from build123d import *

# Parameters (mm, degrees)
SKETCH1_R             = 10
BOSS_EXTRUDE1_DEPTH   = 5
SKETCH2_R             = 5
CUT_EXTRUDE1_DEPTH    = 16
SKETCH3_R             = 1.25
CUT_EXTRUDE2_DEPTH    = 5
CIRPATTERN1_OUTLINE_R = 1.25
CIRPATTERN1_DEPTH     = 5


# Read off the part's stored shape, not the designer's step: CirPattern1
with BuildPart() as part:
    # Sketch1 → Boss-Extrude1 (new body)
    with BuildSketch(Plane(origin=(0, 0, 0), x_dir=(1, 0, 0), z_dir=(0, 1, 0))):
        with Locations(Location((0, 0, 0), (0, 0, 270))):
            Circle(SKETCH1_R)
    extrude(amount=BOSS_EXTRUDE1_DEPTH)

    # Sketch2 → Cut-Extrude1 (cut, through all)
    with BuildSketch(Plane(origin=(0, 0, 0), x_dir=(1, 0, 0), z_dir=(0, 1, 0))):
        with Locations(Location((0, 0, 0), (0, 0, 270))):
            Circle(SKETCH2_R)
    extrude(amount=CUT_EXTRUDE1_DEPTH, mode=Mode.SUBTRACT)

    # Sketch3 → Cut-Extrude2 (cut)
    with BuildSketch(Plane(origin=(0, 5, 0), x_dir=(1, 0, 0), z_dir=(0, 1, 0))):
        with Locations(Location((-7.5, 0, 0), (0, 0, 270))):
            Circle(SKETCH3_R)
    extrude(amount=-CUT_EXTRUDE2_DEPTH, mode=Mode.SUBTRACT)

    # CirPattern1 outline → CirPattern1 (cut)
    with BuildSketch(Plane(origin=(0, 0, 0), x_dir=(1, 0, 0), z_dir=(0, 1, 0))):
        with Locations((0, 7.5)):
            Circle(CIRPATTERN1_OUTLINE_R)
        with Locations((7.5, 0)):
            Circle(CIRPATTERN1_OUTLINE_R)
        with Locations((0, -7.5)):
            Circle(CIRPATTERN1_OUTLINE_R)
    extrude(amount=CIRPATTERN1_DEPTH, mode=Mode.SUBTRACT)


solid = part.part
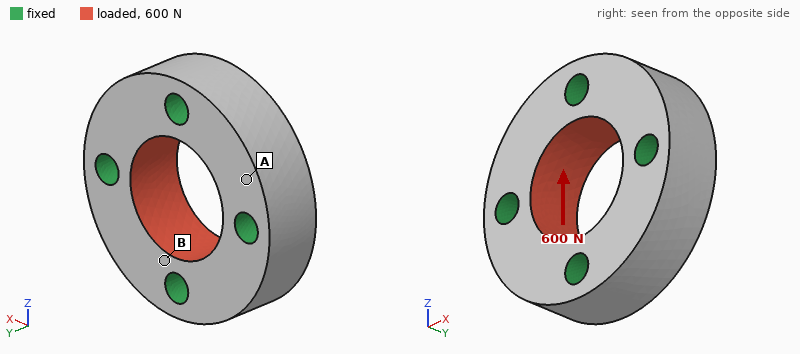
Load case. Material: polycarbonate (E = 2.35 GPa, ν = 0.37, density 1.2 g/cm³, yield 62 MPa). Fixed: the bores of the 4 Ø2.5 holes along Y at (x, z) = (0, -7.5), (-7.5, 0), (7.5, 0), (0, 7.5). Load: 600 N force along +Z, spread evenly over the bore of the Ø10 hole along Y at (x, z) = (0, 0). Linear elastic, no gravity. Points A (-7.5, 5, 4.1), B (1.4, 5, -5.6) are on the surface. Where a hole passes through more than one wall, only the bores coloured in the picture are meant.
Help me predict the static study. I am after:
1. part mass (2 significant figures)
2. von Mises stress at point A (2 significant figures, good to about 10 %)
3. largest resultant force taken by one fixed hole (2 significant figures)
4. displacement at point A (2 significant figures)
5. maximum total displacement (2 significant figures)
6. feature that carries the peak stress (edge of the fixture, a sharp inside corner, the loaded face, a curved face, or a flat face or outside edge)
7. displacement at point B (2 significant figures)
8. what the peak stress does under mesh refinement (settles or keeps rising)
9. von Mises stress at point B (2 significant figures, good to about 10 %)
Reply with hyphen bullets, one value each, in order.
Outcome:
- 1.3 g
- 2.5 MPa
- 160 N
- 5.2 µm
- 13 µm
- edge of the fixture
- 4.7 µm
- keeps rising
- 6.3 MPa
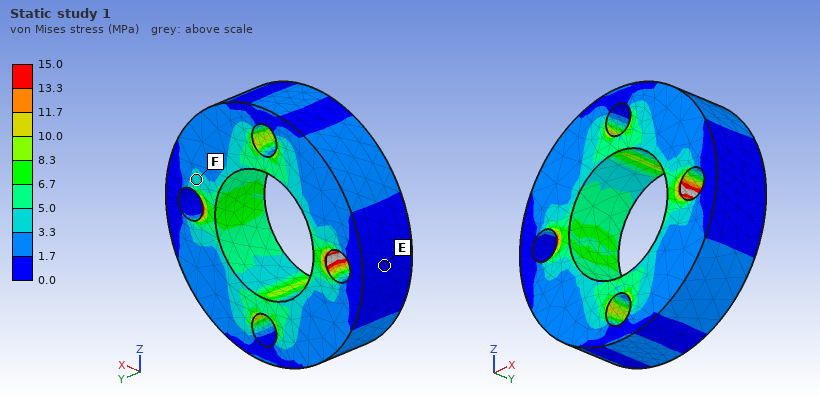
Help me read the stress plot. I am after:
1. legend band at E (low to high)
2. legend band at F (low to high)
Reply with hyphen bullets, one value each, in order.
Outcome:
- 0.0 to 1.7 MPa
- 3.3 to 5.0 MPa
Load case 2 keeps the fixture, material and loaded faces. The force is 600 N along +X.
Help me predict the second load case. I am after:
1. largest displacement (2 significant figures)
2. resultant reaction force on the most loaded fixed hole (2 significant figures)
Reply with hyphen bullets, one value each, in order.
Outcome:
- 13 µm
- 160 N
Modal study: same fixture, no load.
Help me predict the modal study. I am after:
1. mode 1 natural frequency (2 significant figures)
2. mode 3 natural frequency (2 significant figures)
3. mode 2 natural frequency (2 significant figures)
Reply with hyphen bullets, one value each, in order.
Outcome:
- 29 kHz
- 29 kHz
- 29 kHz
